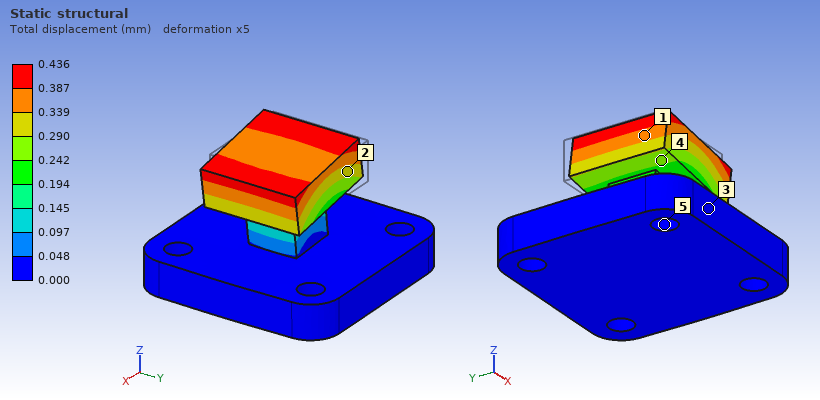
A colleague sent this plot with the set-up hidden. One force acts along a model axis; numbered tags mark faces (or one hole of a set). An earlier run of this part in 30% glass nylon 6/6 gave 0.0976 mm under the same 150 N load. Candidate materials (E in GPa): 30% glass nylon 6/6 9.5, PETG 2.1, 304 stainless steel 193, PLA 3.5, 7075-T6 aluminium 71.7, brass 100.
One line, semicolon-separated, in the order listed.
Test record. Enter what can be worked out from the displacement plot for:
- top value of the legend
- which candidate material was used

0.436 mm; PETG
